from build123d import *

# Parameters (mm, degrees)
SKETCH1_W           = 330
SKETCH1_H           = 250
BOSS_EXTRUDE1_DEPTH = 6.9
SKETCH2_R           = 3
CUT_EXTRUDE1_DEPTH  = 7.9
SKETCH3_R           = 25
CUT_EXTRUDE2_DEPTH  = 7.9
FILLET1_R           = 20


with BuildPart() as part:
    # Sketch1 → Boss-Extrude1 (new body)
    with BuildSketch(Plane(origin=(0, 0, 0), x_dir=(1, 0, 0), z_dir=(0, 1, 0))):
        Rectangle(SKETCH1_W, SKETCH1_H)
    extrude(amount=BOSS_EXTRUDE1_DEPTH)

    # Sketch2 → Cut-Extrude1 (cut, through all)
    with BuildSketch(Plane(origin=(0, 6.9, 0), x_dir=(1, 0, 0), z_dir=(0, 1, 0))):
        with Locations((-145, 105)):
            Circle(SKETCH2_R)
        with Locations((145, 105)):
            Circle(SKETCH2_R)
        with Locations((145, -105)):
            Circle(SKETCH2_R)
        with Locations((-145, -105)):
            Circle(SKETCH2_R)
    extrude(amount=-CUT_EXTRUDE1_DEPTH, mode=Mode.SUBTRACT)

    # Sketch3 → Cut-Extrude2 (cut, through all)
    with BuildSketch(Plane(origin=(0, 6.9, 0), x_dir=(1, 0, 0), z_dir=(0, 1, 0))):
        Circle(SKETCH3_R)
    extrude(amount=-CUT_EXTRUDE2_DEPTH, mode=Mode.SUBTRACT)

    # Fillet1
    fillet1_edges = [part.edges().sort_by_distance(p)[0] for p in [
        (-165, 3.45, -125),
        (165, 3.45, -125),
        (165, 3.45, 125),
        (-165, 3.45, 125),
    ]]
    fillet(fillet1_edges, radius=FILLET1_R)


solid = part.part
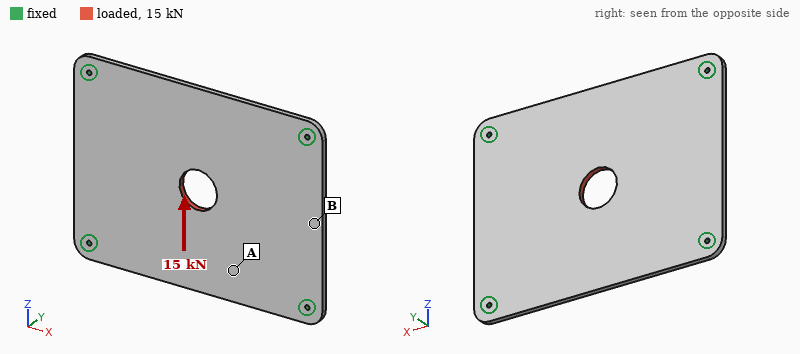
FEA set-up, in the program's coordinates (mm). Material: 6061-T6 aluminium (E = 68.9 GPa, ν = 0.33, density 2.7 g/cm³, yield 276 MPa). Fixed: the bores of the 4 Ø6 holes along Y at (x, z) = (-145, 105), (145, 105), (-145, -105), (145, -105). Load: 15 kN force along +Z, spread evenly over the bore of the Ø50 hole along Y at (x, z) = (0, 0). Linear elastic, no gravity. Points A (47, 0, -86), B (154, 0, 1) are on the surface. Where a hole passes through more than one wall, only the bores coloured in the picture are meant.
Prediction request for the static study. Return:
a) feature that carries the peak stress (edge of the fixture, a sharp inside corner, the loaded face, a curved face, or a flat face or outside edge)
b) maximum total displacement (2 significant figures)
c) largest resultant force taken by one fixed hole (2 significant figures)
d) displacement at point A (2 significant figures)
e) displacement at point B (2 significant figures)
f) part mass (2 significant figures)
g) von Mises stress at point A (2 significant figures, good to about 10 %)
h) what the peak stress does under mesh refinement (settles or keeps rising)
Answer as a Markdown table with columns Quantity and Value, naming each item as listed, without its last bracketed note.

| Quantity | Value |
|---|---|
| feature that carries the peak stress | edge of the fixture |
| maximum total displacement | 40 µm |
| largest resultant force taken by one fixed hole | 4.5 kN |
| displacement at point A | 29 µm |
| displacement at point B | 9.8 µm |
| part mass | 1.5 kg |
| von Mises stress at point A | 6.4 MPa |
| what the peak stress does under mesh refinement | keeps rising |
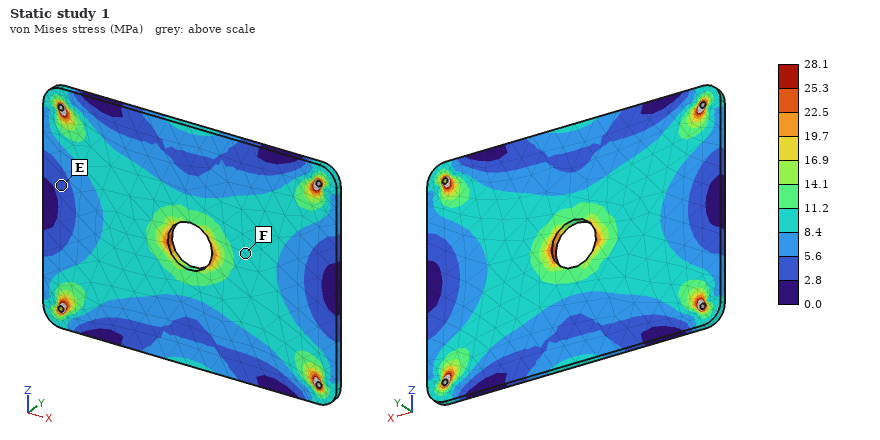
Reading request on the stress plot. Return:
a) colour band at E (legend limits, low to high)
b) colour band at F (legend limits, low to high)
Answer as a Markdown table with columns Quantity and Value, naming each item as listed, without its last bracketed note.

| Quantity | Value |
|---|---|
| colour band at E | 2.8 to 5.6 MPa |
| colour band at F | 8.4 to 11.2 MPa |
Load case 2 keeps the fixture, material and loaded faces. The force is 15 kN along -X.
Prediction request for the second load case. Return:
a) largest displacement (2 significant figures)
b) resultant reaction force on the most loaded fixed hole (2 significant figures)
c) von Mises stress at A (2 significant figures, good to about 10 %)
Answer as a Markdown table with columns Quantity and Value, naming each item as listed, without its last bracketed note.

| Quantity | Value |
|---|---|
| largest displacement | 28 µm |
| resultant reaction force on the most loaded fixed hole | 4.0 kN |
| von Mises stress at A | 4.9 MPa |
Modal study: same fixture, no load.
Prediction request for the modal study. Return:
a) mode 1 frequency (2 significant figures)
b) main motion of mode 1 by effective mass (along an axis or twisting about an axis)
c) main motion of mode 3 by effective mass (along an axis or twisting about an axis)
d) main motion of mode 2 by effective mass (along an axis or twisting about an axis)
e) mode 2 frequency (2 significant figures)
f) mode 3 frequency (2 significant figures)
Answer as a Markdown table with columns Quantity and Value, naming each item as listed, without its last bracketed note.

| Quantity | Value |
|---|---|
| mode 1 frequency | 320 Hz |
| main motion of mode 1 by effective mass | along Y |
| main motion of mode 3 by effective mass | twisting about Z |
| main motion of mode 2 by effective mass | twisting about X |
| mode 2 frequency | 510 Hz |
| mode 3 frequency | 720 Hz |
